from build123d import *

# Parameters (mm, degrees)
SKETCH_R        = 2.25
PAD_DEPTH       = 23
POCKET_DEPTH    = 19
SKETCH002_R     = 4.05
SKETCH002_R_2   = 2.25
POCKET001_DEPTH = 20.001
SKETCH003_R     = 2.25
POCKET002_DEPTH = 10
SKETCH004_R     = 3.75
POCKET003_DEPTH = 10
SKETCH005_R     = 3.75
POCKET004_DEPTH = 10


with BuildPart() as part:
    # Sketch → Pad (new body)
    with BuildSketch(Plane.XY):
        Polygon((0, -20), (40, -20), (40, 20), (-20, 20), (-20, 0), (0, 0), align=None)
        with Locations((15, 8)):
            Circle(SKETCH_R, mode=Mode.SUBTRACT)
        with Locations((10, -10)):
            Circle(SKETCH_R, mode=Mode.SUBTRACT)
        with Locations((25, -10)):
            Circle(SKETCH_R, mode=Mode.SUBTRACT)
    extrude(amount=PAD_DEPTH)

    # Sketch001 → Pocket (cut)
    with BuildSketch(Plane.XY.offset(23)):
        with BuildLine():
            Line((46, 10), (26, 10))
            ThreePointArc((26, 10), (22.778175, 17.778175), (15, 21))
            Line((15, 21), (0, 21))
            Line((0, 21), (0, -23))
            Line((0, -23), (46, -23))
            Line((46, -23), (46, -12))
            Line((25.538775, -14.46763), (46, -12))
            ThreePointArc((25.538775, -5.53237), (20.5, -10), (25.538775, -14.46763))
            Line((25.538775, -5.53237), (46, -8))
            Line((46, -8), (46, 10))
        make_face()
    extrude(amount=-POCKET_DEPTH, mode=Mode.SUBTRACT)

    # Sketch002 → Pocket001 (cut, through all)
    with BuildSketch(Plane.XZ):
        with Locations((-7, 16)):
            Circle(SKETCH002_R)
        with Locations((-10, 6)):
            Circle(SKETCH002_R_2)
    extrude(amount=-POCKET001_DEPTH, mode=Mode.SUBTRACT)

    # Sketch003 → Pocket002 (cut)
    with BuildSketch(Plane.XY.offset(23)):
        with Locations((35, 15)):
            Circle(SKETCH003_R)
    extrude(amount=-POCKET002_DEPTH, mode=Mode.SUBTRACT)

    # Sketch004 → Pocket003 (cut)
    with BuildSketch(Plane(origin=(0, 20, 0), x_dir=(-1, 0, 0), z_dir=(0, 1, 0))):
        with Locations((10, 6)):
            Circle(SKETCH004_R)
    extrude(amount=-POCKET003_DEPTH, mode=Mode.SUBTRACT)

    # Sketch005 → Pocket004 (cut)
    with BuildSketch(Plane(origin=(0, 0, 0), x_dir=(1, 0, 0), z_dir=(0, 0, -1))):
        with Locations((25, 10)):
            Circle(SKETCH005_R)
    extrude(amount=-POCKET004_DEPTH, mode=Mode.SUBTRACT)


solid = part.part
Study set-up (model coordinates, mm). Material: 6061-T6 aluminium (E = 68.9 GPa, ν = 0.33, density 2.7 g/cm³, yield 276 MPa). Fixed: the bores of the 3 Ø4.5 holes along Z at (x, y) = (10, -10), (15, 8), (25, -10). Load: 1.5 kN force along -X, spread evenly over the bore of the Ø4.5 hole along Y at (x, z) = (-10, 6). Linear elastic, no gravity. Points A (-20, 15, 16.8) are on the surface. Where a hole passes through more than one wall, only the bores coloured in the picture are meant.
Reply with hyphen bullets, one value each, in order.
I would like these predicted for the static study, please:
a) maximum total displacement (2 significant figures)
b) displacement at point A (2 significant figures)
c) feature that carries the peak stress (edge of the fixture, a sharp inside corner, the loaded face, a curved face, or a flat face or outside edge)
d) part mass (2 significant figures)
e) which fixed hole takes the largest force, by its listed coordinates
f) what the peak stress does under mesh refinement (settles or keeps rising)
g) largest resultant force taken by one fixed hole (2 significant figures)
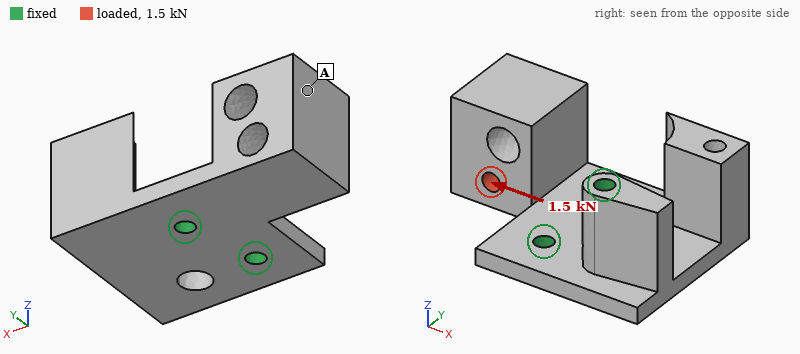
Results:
- 0.33 mm
- 0.29 mm
- a sharp inside corner
- 51 g
- (15, 8)
- keeps rising
- 1.2 kN
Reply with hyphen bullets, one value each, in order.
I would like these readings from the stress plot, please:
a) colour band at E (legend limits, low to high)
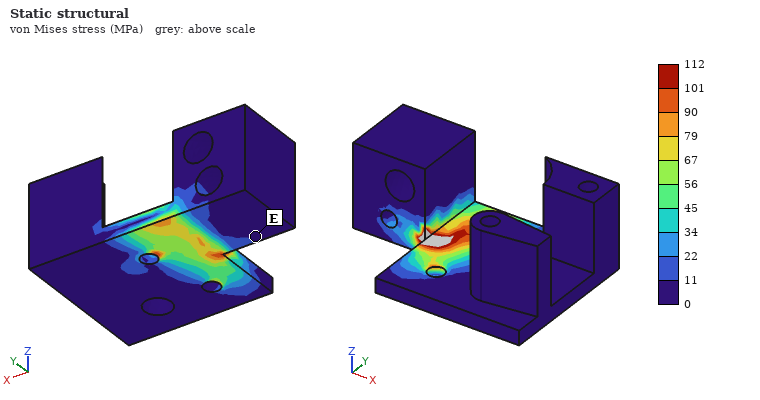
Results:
- 0 to 11 MPa
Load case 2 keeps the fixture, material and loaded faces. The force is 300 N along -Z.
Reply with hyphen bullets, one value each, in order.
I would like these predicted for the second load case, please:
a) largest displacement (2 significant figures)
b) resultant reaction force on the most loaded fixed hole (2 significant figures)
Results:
- 0.26 mm
- 190 N
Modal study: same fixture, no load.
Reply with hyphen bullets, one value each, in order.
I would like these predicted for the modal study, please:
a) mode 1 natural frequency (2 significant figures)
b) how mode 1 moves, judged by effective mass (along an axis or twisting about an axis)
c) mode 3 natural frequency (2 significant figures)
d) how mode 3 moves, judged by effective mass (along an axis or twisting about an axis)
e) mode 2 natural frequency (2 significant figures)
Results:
- 1300 Hz
- along Z
- 3300 Hz
- along Y
- 3000 Hz
